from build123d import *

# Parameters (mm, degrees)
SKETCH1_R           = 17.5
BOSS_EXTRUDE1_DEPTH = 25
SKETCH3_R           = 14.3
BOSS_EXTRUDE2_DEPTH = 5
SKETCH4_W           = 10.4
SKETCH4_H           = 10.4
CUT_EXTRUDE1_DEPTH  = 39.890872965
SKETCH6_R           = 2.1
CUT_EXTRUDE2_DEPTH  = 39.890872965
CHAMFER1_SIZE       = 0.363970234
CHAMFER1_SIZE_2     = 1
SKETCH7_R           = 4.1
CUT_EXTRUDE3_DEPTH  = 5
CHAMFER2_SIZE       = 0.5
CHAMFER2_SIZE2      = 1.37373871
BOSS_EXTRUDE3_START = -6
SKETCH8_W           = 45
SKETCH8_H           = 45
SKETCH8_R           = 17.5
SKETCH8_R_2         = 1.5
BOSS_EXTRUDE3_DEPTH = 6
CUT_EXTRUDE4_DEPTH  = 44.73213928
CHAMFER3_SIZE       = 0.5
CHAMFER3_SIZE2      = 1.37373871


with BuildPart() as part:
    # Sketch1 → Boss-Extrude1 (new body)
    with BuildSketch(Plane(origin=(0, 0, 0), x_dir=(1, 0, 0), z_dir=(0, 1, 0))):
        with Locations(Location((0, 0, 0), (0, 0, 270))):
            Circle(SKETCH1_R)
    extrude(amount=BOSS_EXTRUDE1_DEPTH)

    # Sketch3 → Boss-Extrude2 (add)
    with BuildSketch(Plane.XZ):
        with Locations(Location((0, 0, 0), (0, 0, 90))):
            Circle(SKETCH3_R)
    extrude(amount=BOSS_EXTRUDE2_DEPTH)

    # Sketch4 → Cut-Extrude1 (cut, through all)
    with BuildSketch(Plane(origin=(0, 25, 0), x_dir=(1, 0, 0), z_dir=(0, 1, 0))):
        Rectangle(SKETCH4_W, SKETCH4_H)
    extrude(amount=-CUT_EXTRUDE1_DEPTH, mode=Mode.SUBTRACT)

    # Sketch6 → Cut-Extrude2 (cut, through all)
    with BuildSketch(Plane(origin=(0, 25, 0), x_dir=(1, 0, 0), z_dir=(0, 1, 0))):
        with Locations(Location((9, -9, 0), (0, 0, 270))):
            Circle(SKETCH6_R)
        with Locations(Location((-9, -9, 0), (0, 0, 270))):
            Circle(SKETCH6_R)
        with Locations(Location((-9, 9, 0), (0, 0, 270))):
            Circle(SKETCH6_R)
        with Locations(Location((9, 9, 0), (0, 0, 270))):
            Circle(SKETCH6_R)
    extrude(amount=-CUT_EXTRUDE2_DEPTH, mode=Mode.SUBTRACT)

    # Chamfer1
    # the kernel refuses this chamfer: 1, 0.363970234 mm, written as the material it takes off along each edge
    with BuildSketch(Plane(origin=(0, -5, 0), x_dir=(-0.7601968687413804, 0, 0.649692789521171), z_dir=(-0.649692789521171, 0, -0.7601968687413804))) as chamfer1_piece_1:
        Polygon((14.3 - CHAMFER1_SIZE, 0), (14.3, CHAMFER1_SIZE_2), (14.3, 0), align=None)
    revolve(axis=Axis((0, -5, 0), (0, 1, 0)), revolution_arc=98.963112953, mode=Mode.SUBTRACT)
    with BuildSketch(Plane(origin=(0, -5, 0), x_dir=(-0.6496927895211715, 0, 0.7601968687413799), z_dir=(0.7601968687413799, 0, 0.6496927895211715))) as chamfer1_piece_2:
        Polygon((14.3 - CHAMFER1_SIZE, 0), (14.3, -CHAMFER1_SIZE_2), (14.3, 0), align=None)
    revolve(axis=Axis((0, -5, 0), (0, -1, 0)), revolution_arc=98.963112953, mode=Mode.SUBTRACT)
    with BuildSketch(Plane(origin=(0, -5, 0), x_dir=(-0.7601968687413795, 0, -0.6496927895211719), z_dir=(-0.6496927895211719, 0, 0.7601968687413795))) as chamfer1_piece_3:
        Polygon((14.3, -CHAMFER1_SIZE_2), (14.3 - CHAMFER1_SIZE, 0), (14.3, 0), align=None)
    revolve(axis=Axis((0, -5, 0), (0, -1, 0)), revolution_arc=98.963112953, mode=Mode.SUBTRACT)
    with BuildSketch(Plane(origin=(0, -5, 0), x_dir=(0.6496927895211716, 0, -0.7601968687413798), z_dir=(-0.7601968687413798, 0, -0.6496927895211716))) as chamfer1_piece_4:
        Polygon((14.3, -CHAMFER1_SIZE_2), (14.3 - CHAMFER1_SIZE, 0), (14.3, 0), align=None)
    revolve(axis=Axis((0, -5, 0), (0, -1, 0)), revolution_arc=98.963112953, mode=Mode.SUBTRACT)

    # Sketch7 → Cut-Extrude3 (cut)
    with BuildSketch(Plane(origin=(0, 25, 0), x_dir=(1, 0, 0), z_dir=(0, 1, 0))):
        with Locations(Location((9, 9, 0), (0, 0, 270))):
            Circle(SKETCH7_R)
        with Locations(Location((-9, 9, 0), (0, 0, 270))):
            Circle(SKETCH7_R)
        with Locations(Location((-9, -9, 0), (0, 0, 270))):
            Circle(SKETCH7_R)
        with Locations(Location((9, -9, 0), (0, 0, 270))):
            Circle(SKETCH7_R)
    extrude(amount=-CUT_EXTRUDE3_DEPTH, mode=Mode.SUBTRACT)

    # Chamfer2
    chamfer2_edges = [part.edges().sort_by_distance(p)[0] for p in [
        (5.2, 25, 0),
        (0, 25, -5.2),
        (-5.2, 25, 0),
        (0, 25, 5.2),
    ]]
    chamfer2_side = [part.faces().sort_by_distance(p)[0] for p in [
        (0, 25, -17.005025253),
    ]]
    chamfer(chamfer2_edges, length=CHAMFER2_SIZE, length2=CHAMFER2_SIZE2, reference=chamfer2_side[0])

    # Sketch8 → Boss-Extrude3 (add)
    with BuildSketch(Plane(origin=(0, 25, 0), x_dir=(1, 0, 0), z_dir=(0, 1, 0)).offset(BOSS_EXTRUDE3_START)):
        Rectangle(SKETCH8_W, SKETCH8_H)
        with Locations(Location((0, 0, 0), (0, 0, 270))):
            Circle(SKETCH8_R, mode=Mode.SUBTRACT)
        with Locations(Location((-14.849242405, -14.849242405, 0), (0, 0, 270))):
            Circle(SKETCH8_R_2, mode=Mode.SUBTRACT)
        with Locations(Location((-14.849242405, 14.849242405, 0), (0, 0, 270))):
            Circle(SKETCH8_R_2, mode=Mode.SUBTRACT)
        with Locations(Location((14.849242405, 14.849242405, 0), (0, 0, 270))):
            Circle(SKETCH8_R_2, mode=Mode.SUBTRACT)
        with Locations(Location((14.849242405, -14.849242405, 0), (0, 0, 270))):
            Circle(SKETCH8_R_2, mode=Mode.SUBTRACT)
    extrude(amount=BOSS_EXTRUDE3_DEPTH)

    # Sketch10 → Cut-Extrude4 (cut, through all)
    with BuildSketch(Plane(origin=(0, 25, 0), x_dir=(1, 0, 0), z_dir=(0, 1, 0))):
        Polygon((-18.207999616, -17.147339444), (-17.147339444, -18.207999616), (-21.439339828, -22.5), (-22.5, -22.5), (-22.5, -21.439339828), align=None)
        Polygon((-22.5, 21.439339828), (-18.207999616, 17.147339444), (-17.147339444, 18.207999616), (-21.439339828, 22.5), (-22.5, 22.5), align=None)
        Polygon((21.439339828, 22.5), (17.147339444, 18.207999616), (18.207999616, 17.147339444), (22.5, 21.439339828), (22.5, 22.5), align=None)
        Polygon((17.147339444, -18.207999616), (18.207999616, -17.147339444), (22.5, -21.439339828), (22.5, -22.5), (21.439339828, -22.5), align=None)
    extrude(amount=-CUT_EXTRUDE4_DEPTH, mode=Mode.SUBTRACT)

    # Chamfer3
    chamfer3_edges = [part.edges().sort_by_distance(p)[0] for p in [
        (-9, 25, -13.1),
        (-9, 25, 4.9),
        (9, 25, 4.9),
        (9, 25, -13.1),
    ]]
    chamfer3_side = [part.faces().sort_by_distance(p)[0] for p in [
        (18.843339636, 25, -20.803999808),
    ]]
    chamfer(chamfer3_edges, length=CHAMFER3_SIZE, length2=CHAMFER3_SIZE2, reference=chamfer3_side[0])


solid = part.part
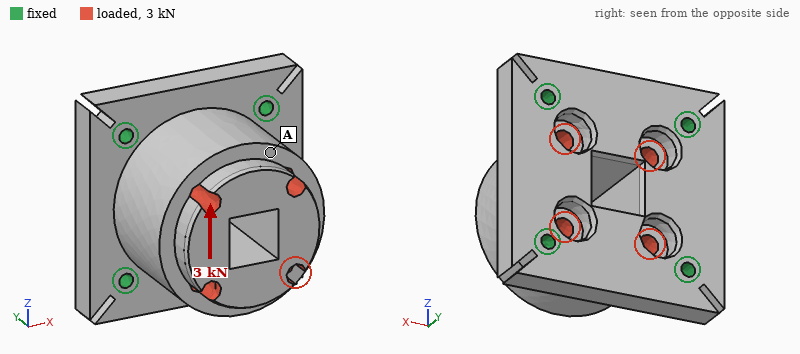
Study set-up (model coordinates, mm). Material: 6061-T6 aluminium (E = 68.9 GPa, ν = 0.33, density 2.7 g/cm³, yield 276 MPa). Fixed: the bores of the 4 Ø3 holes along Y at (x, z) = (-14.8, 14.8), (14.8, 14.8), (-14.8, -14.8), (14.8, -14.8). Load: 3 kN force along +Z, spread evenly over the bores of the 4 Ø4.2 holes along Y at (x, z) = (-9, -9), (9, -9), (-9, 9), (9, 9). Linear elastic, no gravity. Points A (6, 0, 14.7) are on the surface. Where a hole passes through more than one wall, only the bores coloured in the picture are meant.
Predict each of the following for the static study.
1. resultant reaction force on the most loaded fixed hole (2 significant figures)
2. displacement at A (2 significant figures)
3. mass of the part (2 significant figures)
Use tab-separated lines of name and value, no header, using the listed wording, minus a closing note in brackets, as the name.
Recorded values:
resultant reaction force on the most loaded fixed hole	1.0 kN
displacement at A	11 µm
mass of the part	74 g
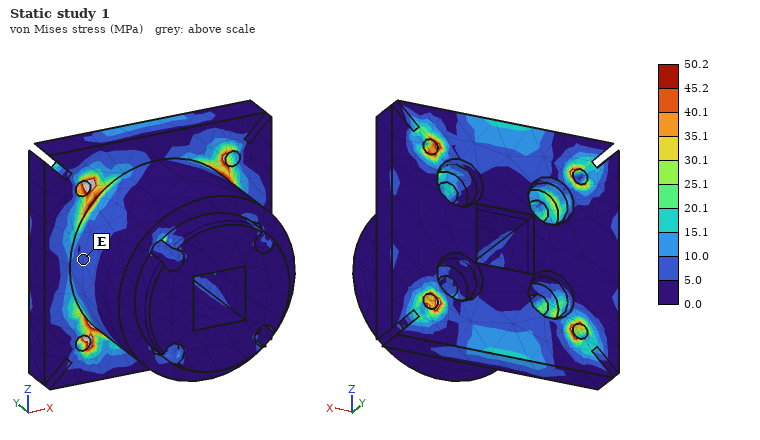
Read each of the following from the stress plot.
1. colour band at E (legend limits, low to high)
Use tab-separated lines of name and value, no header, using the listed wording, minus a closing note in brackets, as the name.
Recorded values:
colour band at E	5.0 to 10.0 MPa
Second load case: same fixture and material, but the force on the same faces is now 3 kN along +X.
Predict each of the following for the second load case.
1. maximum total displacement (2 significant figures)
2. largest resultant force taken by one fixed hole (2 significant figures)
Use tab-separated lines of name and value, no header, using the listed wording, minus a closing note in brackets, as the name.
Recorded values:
maximum total displacement	13 µm
largest resultant force taken by one fixed hole	1.0 kN
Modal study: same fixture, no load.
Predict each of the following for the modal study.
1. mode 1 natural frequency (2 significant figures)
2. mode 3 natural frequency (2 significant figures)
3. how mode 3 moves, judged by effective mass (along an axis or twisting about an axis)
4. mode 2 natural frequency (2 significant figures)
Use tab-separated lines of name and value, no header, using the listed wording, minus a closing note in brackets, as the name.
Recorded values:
mode 1 natural frequency	13 kHz
mode 3 natural frequency	16 kHz
how mode 3 moves, judged by effective mass	along Y
mode 2 natural frequency	13 kHz
